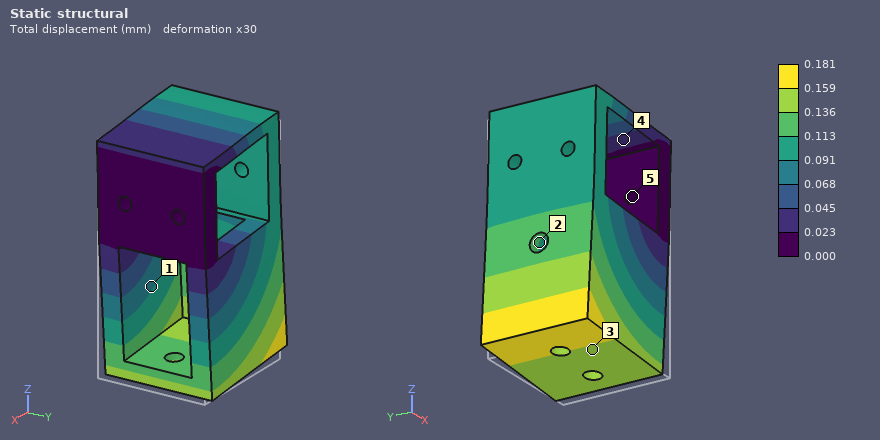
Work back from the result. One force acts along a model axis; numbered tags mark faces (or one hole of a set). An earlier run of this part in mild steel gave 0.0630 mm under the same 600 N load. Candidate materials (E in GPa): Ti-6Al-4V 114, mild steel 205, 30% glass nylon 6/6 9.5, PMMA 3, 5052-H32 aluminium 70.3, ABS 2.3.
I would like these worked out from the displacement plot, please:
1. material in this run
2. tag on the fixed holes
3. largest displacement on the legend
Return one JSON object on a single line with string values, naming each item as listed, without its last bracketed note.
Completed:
{"material in this run": "5052-H32 aluminium", "tag on the fixed holes": "5", "largest displacement on the legend": "0.181 mm"}
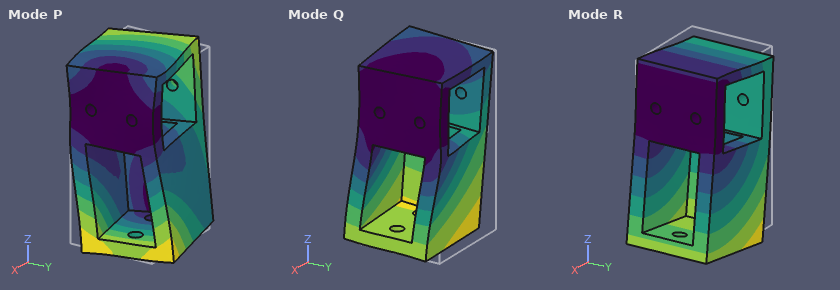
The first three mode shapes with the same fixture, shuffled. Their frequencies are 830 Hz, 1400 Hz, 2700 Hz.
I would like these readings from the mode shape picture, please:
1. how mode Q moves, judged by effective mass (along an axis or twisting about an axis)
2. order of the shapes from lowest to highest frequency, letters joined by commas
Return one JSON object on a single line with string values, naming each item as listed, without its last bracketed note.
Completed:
{"how mode Q moves, judged by effective mass": "along Y", "order of the shapes from lowest to highest frequency, letters joined by commas": "R, Q, P"}
